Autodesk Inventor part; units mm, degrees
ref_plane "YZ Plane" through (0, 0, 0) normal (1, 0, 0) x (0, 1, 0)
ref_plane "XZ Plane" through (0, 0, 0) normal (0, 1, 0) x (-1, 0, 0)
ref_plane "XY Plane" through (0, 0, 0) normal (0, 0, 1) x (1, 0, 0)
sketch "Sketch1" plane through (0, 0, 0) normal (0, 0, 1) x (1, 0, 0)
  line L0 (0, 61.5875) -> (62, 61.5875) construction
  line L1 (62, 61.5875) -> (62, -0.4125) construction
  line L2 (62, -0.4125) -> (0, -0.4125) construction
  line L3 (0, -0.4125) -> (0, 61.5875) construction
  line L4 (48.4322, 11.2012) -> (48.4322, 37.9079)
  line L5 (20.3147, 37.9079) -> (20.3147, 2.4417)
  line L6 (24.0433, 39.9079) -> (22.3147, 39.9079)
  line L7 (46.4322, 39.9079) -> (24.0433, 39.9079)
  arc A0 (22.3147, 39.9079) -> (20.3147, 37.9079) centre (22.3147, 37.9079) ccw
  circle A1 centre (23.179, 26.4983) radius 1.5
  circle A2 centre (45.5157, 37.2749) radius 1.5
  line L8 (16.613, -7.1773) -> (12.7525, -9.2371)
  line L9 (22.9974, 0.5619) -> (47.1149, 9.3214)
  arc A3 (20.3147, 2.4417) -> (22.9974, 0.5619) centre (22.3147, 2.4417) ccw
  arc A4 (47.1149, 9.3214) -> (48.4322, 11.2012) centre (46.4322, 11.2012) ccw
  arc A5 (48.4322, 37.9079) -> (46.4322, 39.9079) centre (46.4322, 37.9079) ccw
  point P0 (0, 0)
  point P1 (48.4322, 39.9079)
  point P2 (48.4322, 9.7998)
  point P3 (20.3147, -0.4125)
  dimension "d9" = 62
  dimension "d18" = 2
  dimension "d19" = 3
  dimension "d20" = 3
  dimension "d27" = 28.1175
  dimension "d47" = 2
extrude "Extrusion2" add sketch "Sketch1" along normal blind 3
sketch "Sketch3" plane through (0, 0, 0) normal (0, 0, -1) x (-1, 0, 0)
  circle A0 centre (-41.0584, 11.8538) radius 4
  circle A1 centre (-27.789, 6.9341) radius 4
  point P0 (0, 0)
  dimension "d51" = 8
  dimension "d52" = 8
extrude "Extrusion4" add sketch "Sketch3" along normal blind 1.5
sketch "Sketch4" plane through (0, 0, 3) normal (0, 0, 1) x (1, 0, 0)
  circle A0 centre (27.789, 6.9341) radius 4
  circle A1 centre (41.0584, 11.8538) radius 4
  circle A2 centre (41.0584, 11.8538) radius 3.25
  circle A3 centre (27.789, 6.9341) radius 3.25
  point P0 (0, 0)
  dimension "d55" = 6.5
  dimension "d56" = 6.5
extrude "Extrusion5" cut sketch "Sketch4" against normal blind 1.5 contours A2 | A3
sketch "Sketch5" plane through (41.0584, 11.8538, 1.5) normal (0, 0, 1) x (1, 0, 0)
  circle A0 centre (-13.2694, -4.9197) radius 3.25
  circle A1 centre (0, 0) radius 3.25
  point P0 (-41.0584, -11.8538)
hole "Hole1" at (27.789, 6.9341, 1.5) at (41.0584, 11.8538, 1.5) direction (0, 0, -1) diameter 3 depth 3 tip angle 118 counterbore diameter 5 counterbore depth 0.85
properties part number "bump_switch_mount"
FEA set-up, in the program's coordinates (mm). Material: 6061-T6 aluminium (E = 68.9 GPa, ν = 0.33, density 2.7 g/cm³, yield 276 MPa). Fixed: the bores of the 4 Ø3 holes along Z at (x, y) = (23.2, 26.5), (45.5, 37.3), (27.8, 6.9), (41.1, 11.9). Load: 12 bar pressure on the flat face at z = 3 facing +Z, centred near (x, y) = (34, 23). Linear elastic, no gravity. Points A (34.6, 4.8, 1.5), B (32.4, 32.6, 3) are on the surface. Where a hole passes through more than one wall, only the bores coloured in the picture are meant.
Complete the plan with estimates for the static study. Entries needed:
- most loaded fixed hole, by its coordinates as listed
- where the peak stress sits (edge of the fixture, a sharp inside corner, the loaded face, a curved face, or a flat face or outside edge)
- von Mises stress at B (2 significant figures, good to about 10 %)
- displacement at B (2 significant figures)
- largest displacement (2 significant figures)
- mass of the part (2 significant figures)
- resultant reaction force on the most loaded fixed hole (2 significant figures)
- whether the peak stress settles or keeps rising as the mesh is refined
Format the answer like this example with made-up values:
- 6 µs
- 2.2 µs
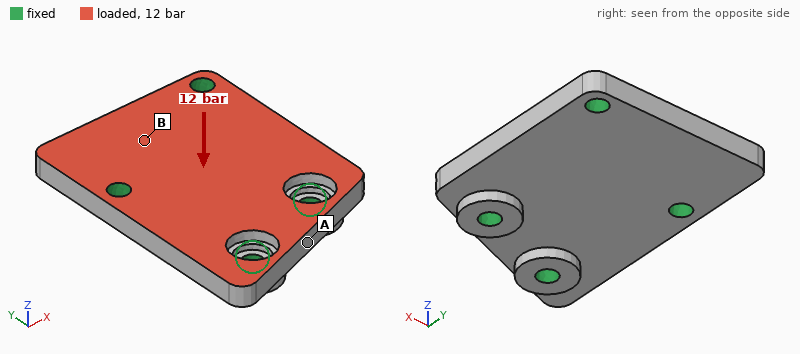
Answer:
- (23.2, 26.5)
- edge of the fixture
- 24 MPa
- 11 µm
- 21 µm
- 7.8 g
- 380 N
- keeps rising
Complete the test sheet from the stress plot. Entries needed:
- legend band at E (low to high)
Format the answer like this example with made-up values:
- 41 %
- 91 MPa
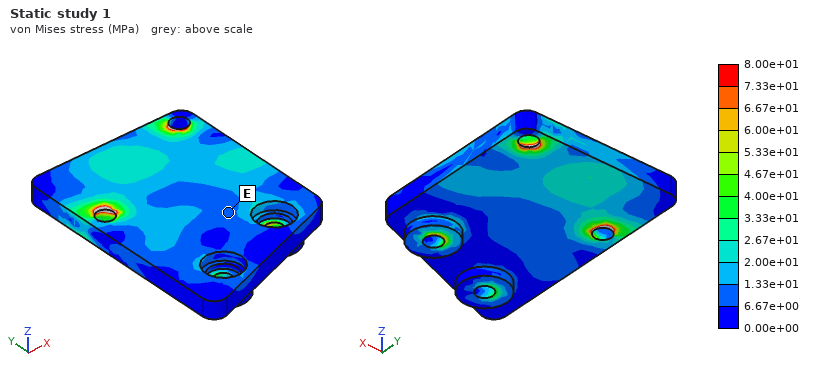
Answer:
- 6.67e+00 to 1.33e+01 MPa
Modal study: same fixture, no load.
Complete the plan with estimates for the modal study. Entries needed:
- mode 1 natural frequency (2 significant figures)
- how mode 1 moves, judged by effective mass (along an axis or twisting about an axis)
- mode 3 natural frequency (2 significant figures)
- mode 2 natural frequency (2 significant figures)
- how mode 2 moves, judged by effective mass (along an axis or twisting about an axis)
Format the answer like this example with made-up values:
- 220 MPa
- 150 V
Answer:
- 17 kHz
- along Z
- 29 kHz
- 22 kHz
- along Z
